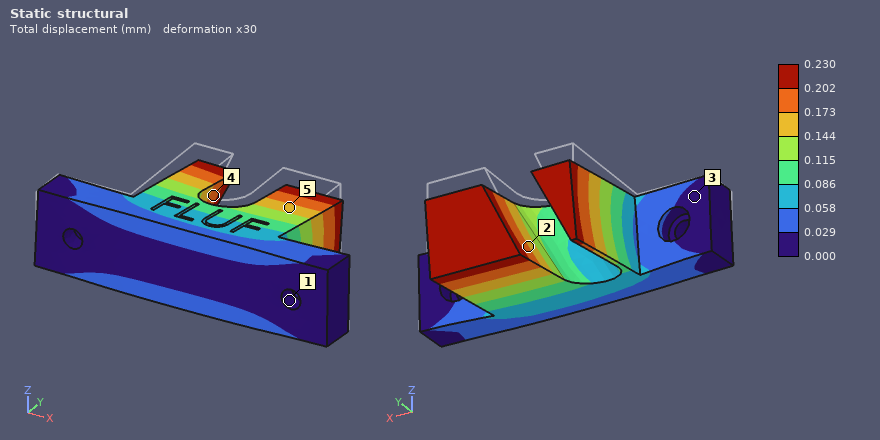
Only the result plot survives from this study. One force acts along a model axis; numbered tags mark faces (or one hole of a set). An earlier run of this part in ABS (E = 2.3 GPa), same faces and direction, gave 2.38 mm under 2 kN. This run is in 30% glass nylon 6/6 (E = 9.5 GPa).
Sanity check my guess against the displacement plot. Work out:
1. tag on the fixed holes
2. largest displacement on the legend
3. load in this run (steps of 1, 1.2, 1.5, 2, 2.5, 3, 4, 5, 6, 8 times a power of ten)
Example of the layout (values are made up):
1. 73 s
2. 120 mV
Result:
1. 1
2. 0.230 mm
3. 800 N
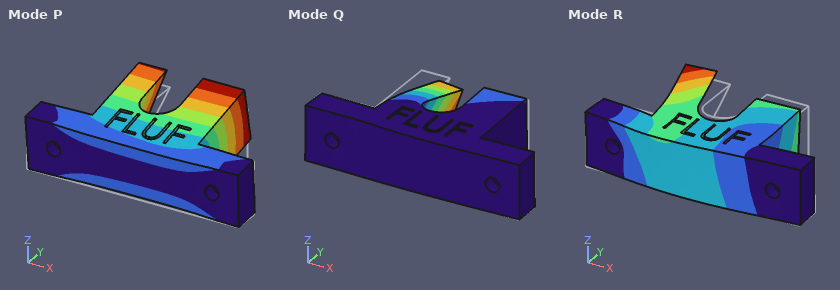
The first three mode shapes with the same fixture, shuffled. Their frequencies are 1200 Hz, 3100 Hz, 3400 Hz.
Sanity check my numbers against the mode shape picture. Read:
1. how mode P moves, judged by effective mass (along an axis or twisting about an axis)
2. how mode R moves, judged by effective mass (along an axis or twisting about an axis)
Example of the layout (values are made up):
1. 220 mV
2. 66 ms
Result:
1. along Z
2. along Y
